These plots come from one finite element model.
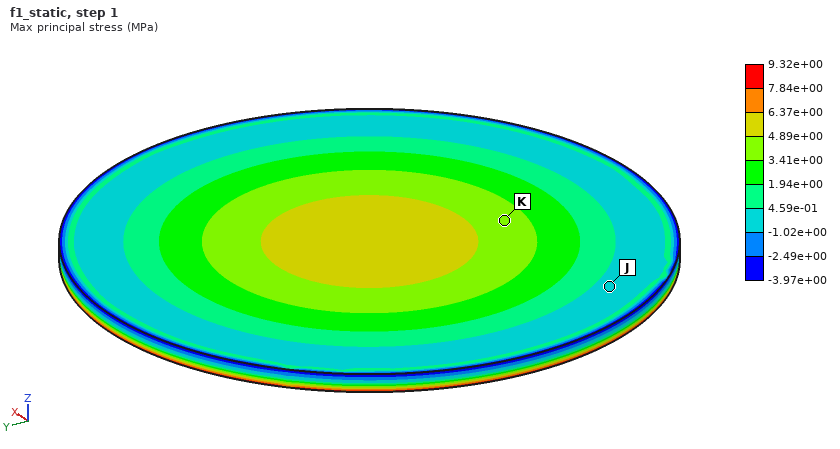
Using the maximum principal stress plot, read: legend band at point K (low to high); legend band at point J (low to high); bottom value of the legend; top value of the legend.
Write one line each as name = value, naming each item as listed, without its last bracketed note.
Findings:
legend band at point K = 3.41e+00 to 4.89e+00 MPa
legend band at point J = -1.02e+00 to 4.59e-01 MPa
bottom value of the legend = -3.97e+00 MPa
top value of the legend = 9.32e+00 MPa
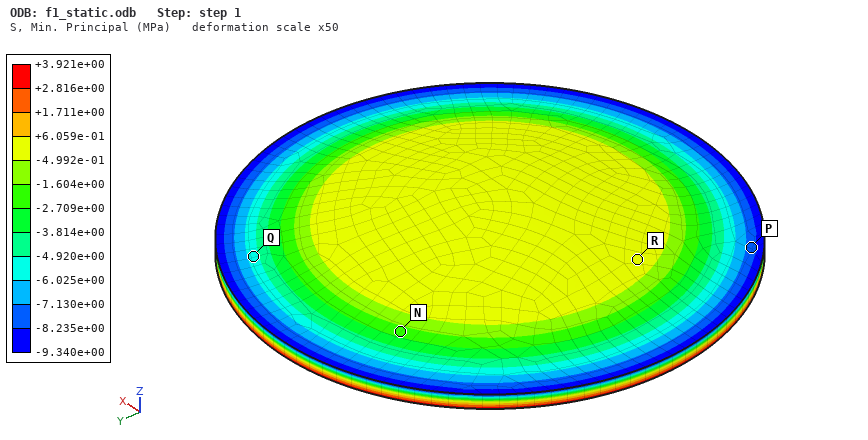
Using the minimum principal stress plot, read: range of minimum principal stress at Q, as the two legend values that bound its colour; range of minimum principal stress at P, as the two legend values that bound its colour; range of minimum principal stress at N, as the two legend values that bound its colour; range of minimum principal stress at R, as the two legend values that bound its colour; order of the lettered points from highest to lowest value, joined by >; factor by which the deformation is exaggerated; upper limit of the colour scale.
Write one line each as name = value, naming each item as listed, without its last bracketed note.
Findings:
range of minimum principal stress at Q, as the two legend values that bound its colour = -6.025e+00 to -4.920e+00 MPa
range of minimum principal stress at P, as the two legend values that bound its colour = -8.235e+00 to -7.130e+00 MPa
range of minimum principal stress at N, as the two legend values that bound its colour = -2.709e+00 to -1.604e+00 MPa
range of minimum principal stress at R, as the two legend values that bound its colour = -4.992e-01 to +6.059e-01 MPa
order of the lettered points from highest to lowest value, joined by > = R > N > Q > P
factor by which the deformation is exaggerated = 50
upper limit of the colour scale = +3.921e+00 MPa
